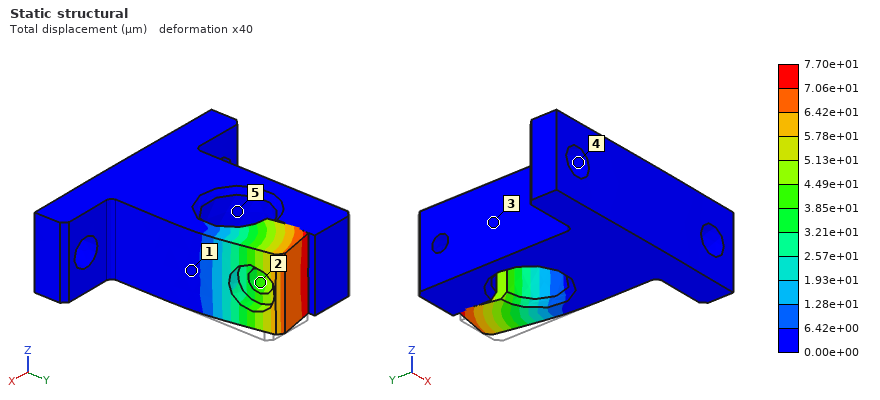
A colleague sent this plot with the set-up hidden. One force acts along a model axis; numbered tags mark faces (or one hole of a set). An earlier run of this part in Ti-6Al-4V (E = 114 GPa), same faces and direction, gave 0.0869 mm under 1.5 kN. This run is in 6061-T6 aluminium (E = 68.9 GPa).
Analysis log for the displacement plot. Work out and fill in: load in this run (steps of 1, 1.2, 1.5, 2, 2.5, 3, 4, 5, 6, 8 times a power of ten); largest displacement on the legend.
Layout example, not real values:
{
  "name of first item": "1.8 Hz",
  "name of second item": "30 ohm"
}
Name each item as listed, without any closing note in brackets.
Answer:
{
  "load in this run": "800 N",
  "largest displacement on the legend": "7.70e+01 µm"
}
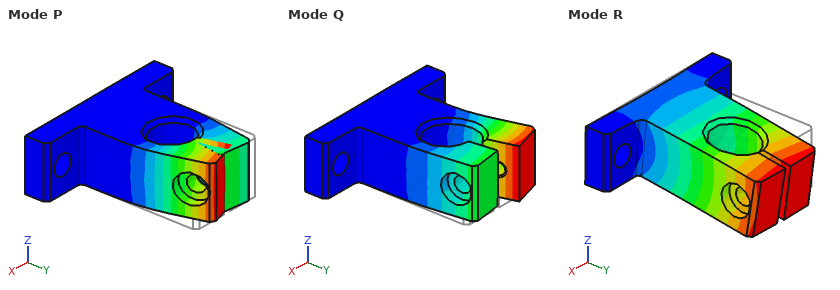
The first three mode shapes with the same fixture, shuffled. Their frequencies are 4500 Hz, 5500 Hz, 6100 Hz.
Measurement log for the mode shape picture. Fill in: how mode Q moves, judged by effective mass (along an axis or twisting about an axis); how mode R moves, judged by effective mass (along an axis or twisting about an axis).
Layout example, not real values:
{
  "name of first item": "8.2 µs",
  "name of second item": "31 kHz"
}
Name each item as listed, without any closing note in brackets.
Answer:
{
  "how mode Q moves, judged by effective mass": "along X",
  "how mode R moves, judged by effective mass": "along Z"
}
